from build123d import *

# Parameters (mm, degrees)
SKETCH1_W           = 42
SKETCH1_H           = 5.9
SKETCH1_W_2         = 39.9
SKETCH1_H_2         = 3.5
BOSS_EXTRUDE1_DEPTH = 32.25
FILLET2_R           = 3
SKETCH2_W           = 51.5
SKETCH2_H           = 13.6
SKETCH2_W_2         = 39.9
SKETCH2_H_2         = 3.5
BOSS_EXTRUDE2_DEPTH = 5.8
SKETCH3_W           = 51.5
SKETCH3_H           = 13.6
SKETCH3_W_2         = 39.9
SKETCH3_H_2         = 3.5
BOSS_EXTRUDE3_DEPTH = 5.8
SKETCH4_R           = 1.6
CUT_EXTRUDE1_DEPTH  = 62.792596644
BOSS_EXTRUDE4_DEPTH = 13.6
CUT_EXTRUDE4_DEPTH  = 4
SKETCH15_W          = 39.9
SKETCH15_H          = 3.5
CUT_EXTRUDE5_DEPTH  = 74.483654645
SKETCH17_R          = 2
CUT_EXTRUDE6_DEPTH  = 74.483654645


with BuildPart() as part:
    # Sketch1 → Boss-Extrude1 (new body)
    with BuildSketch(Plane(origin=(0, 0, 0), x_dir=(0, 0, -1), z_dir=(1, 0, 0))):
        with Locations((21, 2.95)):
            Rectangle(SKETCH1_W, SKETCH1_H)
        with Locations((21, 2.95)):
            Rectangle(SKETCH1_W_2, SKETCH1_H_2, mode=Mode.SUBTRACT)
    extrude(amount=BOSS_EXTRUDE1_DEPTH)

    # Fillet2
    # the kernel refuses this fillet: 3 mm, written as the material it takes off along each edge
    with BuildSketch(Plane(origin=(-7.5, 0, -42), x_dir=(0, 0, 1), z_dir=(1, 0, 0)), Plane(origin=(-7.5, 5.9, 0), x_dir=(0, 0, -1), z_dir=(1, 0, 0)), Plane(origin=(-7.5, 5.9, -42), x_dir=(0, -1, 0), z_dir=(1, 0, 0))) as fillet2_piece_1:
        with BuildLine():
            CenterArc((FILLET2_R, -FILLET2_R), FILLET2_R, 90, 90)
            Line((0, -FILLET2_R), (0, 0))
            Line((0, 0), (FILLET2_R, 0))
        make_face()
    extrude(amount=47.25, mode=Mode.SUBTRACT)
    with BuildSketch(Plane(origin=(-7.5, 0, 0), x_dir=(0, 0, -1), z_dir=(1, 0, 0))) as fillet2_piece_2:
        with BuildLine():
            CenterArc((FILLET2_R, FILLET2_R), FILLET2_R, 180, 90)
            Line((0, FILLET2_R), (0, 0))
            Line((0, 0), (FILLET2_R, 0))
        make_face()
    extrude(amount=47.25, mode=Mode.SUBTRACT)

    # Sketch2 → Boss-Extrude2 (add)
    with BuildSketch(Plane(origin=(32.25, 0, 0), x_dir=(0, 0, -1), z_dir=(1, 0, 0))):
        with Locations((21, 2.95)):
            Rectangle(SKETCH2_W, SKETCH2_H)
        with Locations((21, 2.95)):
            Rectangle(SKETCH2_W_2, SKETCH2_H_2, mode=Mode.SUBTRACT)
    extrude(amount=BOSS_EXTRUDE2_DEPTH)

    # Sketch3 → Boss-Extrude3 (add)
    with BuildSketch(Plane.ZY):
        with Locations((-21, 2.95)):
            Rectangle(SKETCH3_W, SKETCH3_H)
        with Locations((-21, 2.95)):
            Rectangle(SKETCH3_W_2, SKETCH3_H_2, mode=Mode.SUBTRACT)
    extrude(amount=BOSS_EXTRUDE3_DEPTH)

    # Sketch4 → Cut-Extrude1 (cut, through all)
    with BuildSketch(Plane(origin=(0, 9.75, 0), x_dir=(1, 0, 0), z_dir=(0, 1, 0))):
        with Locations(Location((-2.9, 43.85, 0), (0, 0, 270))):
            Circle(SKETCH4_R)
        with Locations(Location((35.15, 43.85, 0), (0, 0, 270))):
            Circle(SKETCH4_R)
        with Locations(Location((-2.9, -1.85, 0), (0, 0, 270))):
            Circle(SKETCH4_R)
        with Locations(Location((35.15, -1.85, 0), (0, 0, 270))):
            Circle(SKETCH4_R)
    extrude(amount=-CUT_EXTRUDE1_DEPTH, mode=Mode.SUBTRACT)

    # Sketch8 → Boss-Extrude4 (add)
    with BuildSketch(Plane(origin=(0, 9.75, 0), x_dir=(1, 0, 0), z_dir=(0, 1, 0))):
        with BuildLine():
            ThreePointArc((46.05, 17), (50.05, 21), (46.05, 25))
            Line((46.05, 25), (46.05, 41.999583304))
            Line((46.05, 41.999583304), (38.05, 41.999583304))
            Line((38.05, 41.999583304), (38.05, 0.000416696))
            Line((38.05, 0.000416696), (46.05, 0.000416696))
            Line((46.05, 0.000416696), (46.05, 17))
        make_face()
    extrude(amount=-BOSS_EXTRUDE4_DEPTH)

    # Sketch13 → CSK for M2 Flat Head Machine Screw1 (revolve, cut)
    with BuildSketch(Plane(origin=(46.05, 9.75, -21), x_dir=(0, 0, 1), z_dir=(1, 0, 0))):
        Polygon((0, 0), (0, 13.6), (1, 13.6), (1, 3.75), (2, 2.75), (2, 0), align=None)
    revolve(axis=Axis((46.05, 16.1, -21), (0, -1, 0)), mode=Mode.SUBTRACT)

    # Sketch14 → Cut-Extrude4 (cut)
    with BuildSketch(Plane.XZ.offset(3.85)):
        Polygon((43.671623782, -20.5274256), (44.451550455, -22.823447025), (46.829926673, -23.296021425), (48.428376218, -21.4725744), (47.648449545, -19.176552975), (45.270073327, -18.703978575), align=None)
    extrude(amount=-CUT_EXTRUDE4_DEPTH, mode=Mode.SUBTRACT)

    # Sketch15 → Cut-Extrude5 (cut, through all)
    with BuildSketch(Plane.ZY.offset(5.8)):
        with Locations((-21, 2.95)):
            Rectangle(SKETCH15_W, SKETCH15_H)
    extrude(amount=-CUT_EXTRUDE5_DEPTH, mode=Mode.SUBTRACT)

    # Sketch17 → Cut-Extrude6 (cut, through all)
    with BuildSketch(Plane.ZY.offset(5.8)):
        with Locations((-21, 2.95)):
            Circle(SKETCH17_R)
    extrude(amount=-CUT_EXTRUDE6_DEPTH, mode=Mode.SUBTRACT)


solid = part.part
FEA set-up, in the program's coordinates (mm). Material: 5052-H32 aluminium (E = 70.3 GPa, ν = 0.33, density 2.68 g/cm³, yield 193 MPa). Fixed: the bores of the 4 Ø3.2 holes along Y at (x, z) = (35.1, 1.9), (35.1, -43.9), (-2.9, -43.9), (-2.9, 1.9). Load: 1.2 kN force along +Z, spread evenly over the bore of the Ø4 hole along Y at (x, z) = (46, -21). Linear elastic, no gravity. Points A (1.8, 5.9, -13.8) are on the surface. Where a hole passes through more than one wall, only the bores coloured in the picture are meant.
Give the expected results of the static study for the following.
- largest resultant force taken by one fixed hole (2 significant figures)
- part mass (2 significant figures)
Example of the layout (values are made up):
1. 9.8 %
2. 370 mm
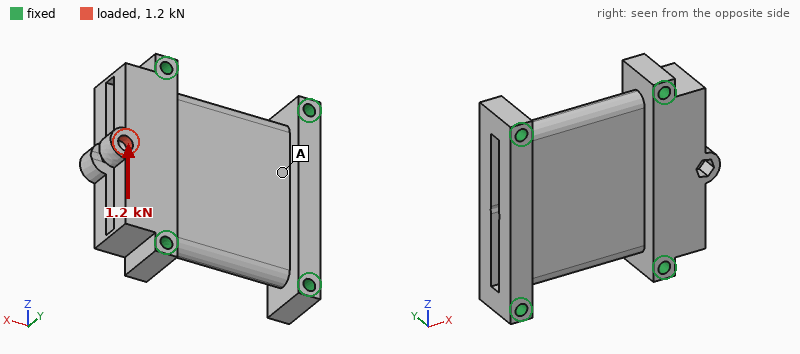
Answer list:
1. 660 N
2. 34 g
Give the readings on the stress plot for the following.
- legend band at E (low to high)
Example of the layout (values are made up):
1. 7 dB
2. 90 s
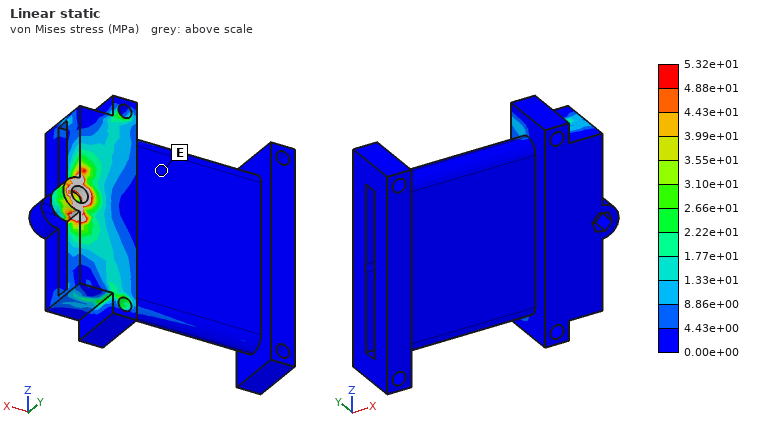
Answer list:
1. 0.00e+00 to 4.43e+00 MPa
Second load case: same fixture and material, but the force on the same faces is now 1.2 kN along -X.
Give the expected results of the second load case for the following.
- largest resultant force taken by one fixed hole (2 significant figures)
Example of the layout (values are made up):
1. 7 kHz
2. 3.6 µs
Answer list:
1. 560 N
